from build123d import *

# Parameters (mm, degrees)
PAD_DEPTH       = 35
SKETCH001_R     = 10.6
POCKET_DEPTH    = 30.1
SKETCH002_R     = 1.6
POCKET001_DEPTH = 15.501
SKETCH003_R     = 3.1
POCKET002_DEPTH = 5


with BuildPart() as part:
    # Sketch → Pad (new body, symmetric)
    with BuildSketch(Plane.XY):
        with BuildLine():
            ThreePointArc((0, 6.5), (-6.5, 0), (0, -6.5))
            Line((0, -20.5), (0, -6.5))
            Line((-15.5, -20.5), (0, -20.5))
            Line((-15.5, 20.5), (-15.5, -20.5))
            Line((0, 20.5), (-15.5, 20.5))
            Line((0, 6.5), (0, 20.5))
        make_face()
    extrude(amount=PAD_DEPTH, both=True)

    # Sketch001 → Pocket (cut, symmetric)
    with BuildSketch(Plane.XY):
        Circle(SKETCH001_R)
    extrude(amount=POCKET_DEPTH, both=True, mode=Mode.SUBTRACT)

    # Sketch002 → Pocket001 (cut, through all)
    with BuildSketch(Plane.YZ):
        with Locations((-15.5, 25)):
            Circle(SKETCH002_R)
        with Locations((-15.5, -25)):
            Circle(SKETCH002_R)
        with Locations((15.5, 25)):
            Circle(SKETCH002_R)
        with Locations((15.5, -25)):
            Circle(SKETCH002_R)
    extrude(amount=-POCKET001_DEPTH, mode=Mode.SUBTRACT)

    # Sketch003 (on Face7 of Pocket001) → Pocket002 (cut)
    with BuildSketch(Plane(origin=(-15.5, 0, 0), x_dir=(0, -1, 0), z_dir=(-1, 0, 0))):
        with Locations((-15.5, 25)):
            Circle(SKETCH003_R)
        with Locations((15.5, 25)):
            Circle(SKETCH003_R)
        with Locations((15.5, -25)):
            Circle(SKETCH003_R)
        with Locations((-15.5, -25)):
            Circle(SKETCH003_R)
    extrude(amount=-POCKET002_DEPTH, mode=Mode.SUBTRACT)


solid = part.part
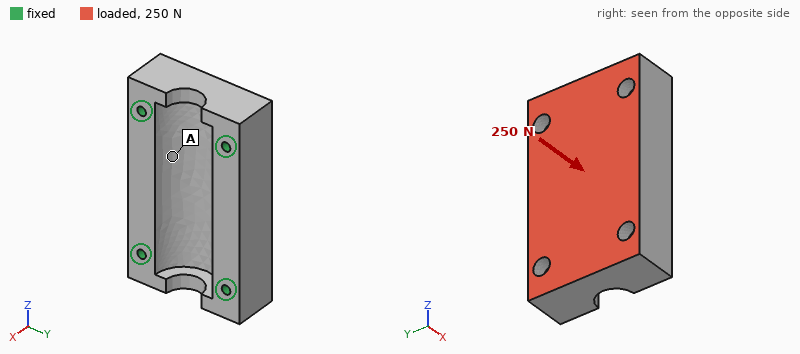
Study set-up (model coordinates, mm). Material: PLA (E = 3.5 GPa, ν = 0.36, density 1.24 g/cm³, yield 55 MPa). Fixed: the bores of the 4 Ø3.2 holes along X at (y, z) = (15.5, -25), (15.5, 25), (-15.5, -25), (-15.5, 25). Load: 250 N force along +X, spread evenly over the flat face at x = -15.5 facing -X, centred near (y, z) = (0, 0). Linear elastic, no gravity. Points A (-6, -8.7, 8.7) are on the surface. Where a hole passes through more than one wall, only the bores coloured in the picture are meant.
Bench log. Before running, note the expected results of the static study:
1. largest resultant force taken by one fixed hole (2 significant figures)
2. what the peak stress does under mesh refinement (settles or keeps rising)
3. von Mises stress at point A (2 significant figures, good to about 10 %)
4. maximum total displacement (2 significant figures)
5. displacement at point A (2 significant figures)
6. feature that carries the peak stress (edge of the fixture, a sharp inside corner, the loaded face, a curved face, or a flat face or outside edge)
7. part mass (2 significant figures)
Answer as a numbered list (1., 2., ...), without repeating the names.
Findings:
1. 71 N
2. keeps rising
3. 0.35 MPa
4. 8.5 µm
5. 6.2 µm
6. edge of the fixture
7. 40 g
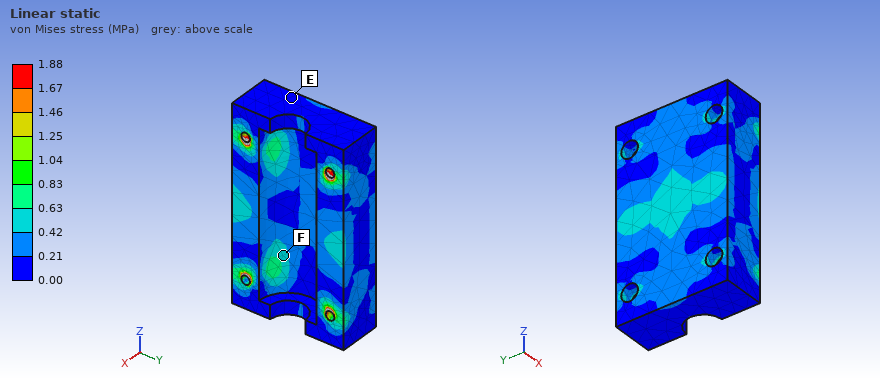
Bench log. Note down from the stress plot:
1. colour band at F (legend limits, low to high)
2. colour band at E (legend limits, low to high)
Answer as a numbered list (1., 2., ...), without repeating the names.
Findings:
1. 0.42 to 0.63 MPa
2. 0.00 to 0.21 MPa
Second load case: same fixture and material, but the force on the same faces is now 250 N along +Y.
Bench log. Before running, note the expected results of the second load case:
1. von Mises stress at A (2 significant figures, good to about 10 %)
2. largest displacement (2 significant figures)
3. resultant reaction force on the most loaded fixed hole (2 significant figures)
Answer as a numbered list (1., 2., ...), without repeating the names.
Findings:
1. 0.26 MPa
2. 6.6 µm
3. 72 N
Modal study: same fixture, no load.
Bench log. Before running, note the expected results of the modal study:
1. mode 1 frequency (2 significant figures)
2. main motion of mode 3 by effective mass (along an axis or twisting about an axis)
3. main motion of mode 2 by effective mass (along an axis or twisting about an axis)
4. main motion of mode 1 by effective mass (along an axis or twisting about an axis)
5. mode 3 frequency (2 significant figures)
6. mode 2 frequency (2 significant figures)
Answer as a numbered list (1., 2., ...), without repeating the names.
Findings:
1. 5500 Hz
2. along Y
3. along Y
4. along X
5. 7500 Hz
6. 5900 Hz
